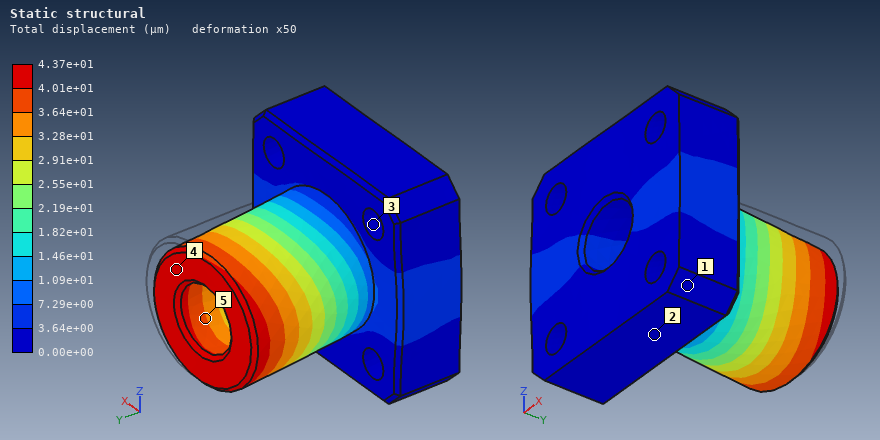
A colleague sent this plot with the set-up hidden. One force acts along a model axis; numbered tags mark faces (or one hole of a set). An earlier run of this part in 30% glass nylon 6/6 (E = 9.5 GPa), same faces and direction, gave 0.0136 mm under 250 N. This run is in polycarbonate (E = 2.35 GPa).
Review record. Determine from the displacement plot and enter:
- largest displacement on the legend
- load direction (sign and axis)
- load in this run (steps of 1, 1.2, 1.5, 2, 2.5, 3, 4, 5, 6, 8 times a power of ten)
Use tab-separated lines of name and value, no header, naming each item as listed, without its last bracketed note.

largest displacement on the legend	4.37e+01 µm
load direction	-X
load in this run	200 N
